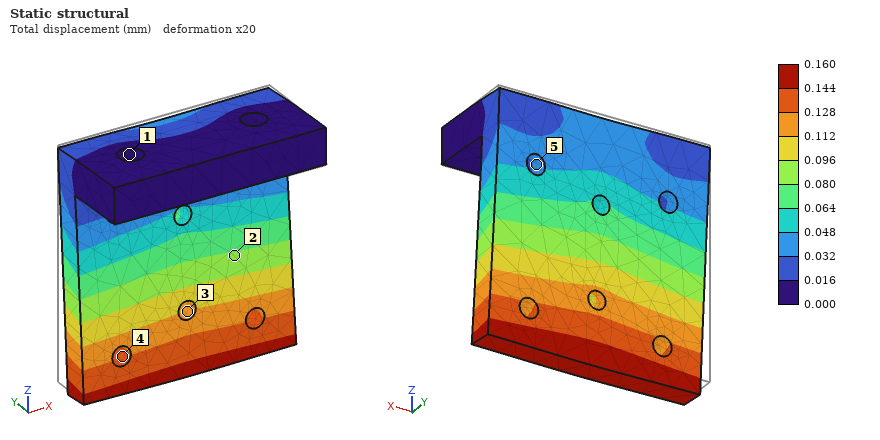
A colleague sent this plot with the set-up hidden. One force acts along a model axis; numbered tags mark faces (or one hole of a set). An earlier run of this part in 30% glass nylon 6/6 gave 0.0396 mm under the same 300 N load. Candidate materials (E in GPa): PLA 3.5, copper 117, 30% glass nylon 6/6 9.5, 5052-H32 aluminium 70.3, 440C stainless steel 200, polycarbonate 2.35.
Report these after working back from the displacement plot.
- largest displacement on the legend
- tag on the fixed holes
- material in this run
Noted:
0.160 mm
1
polycarbonate
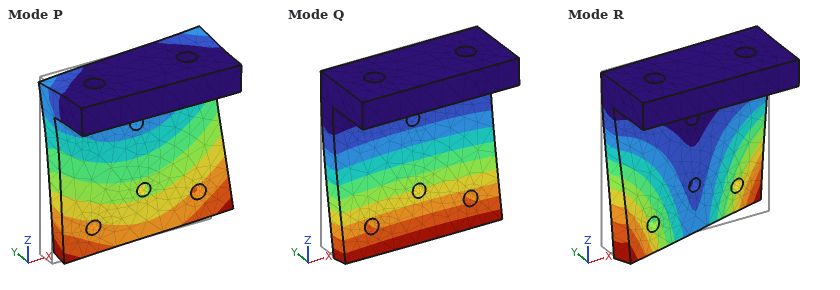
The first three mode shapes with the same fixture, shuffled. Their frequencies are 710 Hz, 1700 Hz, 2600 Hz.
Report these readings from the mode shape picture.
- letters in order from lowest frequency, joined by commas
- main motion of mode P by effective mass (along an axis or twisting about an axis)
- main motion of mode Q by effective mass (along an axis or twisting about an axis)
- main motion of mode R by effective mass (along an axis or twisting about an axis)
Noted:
Q, R, P
along X
along Y
twisting about Z
